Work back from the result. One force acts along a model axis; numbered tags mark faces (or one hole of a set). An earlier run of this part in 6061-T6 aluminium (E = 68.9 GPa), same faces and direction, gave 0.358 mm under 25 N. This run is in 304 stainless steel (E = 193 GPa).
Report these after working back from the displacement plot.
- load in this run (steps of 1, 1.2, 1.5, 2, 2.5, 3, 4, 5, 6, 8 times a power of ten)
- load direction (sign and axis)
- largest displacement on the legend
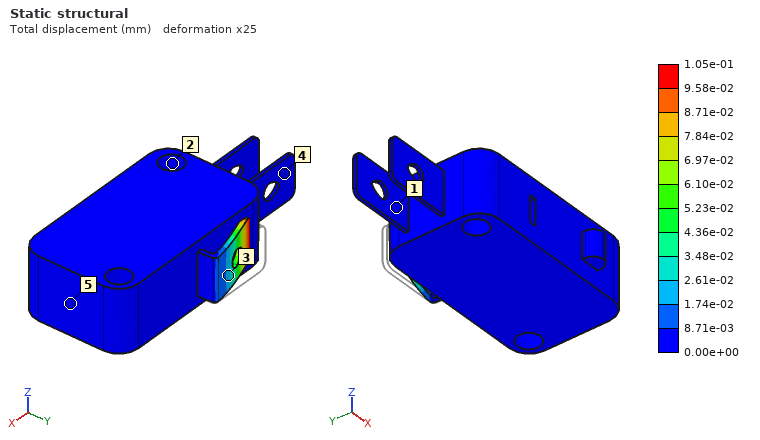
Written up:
20 N
-Y
1.05e-01 mm
